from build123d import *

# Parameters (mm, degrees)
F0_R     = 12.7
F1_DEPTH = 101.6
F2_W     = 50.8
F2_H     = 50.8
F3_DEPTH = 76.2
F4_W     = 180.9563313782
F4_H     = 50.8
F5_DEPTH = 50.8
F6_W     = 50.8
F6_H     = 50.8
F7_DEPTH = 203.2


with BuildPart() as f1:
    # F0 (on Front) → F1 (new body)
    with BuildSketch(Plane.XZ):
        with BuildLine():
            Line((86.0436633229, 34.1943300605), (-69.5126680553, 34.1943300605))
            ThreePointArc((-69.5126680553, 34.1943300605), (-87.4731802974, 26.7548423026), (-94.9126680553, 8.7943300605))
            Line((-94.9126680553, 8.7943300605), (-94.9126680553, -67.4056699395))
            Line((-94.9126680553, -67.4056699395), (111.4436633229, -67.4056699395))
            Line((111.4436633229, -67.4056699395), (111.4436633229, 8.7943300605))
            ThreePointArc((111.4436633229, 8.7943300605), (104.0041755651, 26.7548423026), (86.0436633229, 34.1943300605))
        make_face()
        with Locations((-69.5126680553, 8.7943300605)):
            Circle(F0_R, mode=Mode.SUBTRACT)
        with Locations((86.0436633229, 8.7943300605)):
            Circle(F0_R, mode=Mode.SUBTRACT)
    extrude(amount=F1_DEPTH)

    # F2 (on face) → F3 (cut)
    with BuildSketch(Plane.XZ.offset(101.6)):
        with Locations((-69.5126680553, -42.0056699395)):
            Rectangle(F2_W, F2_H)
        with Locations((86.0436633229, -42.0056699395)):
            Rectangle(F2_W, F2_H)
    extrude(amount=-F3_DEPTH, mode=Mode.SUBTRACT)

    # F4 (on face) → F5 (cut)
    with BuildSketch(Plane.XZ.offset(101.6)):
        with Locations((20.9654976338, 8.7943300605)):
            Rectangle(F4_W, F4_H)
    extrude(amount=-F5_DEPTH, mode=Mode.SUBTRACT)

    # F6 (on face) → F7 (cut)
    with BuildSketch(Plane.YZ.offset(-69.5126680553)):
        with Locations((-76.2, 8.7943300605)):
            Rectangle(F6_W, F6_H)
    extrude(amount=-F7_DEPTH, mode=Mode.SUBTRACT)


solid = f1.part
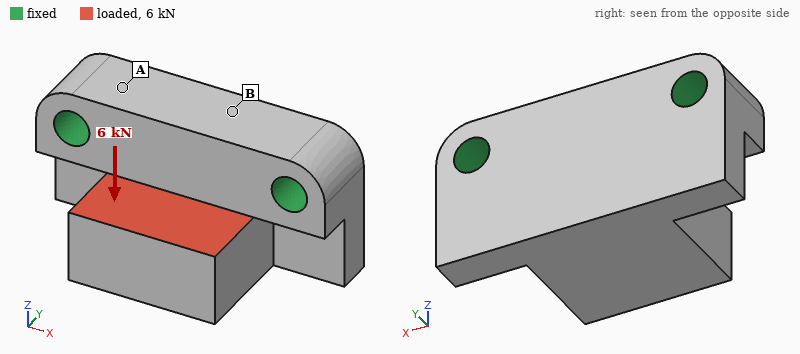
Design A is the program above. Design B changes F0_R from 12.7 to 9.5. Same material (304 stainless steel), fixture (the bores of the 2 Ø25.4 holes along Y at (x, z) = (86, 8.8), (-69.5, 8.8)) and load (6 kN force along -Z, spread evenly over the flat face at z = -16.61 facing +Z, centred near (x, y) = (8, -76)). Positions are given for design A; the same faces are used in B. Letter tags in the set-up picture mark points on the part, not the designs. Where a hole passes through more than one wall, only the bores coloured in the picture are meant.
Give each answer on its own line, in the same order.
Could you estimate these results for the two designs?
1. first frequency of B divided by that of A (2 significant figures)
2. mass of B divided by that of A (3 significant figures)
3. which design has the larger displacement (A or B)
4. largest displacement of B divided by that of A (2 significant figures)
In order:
0.94
1.02
B
1.1
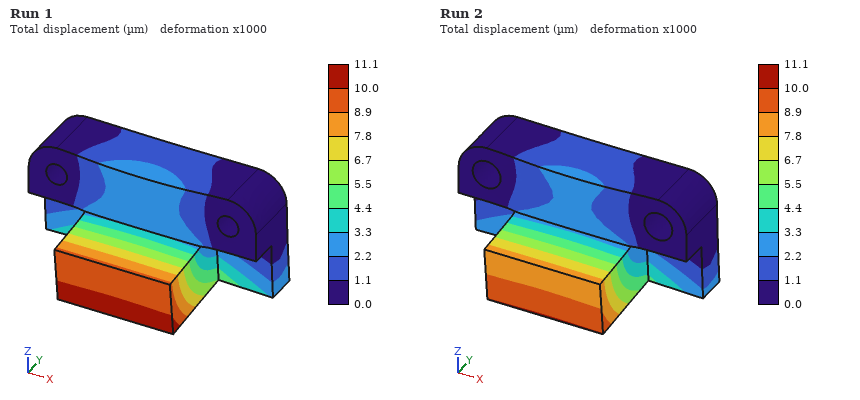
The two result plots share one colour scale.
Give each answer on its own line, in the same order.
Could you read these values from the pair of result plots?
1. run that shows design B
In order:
Run 1
